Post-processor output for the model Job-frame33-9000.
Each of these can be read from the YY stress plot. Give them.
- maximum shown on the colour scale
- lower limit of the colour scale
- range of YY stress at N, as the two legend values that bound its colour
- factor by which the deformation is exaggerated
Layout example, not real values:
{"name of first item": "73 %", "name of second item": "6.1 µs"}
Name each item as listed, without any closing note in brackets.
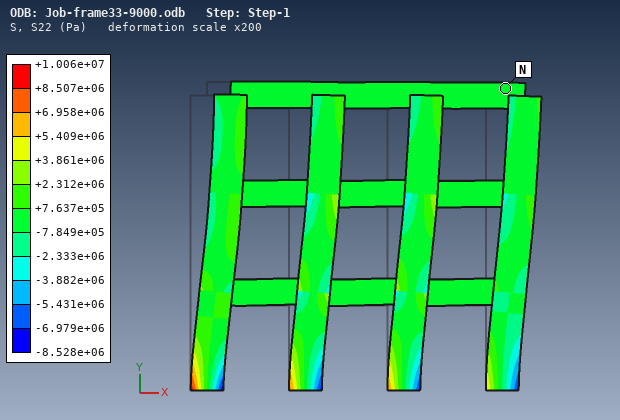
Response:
{"maximum shown on the colour scale": "+1.006e+07 Pa", "lower limit of the colour scale": "-8.528e+06 Pa", "range of YY stress at N, as the two legend values that bound its colour": "-7.849e+05 to +7.637e+05 Pa", "factor by which the deformation is exaggerated": "200"}
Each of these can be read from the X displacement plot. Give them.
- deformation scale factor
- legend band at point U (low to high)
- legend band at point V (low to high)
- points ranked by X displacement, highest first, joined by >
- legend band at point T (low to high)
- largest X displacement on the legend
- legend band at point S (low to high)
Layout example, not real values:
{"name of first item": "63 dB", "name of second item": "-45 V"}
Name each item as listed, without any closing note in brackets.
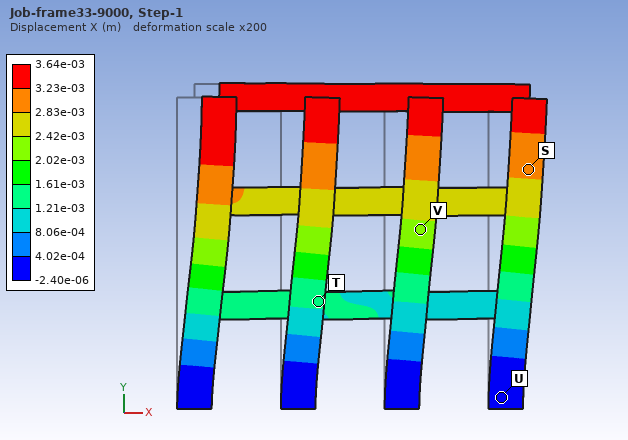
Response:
{"deformation scale factor": "200", "legend band at point U": "-2.40e-06 to 4.02e-04 m", "legend band at point V": "2.02e-03 to 2.42e-03 m", "points ranked by X displacement, highest first, joined by >": "S > V > T > U", "legend band at point T": "1.21e-03 to 1.61e-03 m", "largest X displacement on the legend": "3.64e-03 m", "legend band at point S": "2.83e-03 to 3.23e-03 m"}
